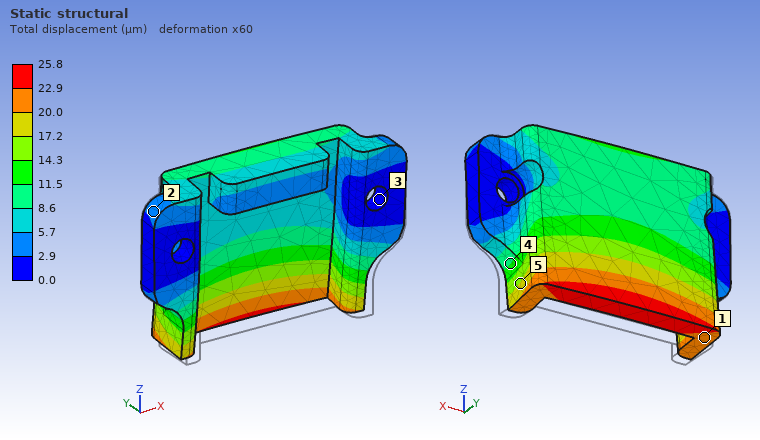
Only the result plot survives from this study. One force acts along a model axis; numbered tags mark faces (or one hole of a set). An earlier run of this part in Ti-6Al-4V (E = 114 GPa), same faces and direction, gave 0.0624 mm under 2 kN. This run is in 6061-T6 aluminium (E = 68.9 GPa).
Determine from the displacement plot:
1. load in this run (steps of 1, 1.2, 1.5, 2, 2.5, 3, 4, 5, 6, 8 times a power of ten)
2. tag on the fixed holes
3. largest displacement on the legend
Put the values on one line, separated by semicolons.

500 N; 3; 25.8 µm
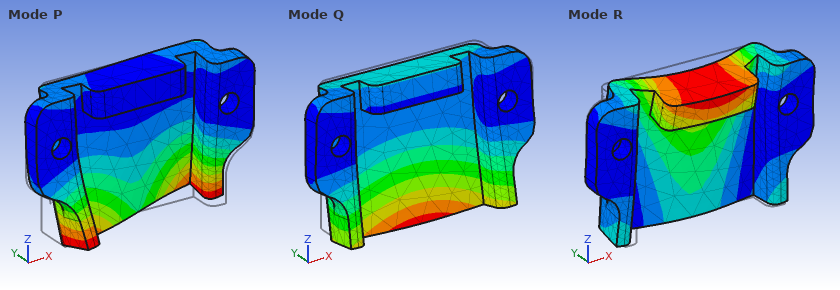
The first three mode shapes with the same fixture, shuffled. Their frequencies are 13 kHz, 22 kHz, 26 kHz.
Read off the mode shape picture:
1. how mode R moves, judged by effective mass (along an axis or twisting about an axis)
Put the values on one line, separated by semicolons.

along Y
